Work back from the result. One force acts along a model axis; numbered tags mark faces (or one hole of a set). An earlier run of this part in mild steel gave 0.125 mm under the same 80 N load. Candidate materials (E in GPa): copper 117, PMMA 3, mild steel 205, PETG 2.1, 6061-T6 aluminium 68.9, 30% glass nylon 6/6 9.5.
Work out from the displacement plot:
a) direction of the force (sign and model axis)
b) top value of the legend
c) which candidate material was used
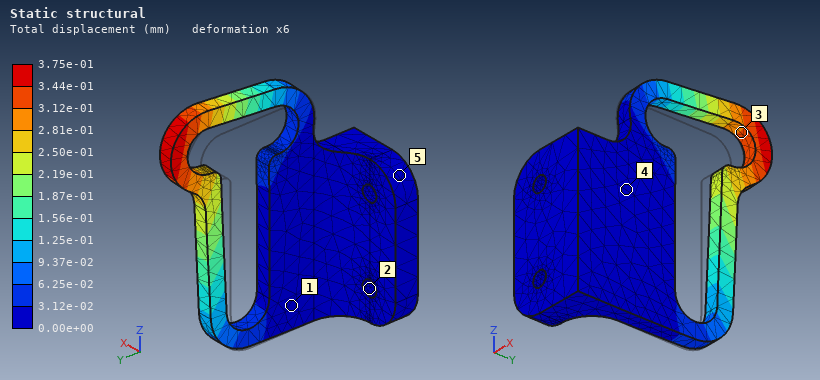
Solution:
+X
3.75e-01 mm
6061-T6 aluminium
